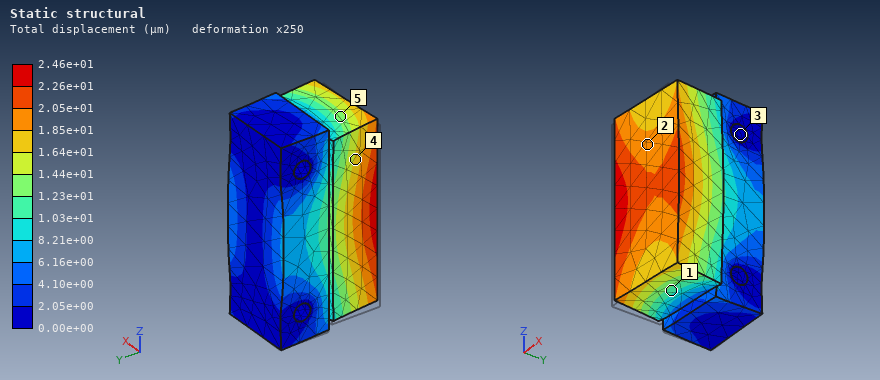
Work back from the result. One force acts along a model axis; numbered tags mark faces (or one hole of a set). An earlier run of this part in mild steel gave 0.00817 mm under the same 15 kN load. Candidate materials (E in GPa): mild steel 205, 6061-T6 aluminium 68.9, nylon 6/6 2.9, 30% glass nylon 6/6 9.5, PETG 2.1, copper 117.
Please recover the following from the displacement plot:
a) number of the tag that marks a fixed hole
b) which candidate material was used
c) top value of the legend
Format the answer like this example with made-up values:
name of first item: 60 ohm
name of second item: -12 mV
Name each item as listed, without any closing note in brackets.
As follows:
number of the tag that marks a fixed hole: 3
which candidate material was used: 6061-T6 aluminium
top value of the legend: 2.46e+01 µm
